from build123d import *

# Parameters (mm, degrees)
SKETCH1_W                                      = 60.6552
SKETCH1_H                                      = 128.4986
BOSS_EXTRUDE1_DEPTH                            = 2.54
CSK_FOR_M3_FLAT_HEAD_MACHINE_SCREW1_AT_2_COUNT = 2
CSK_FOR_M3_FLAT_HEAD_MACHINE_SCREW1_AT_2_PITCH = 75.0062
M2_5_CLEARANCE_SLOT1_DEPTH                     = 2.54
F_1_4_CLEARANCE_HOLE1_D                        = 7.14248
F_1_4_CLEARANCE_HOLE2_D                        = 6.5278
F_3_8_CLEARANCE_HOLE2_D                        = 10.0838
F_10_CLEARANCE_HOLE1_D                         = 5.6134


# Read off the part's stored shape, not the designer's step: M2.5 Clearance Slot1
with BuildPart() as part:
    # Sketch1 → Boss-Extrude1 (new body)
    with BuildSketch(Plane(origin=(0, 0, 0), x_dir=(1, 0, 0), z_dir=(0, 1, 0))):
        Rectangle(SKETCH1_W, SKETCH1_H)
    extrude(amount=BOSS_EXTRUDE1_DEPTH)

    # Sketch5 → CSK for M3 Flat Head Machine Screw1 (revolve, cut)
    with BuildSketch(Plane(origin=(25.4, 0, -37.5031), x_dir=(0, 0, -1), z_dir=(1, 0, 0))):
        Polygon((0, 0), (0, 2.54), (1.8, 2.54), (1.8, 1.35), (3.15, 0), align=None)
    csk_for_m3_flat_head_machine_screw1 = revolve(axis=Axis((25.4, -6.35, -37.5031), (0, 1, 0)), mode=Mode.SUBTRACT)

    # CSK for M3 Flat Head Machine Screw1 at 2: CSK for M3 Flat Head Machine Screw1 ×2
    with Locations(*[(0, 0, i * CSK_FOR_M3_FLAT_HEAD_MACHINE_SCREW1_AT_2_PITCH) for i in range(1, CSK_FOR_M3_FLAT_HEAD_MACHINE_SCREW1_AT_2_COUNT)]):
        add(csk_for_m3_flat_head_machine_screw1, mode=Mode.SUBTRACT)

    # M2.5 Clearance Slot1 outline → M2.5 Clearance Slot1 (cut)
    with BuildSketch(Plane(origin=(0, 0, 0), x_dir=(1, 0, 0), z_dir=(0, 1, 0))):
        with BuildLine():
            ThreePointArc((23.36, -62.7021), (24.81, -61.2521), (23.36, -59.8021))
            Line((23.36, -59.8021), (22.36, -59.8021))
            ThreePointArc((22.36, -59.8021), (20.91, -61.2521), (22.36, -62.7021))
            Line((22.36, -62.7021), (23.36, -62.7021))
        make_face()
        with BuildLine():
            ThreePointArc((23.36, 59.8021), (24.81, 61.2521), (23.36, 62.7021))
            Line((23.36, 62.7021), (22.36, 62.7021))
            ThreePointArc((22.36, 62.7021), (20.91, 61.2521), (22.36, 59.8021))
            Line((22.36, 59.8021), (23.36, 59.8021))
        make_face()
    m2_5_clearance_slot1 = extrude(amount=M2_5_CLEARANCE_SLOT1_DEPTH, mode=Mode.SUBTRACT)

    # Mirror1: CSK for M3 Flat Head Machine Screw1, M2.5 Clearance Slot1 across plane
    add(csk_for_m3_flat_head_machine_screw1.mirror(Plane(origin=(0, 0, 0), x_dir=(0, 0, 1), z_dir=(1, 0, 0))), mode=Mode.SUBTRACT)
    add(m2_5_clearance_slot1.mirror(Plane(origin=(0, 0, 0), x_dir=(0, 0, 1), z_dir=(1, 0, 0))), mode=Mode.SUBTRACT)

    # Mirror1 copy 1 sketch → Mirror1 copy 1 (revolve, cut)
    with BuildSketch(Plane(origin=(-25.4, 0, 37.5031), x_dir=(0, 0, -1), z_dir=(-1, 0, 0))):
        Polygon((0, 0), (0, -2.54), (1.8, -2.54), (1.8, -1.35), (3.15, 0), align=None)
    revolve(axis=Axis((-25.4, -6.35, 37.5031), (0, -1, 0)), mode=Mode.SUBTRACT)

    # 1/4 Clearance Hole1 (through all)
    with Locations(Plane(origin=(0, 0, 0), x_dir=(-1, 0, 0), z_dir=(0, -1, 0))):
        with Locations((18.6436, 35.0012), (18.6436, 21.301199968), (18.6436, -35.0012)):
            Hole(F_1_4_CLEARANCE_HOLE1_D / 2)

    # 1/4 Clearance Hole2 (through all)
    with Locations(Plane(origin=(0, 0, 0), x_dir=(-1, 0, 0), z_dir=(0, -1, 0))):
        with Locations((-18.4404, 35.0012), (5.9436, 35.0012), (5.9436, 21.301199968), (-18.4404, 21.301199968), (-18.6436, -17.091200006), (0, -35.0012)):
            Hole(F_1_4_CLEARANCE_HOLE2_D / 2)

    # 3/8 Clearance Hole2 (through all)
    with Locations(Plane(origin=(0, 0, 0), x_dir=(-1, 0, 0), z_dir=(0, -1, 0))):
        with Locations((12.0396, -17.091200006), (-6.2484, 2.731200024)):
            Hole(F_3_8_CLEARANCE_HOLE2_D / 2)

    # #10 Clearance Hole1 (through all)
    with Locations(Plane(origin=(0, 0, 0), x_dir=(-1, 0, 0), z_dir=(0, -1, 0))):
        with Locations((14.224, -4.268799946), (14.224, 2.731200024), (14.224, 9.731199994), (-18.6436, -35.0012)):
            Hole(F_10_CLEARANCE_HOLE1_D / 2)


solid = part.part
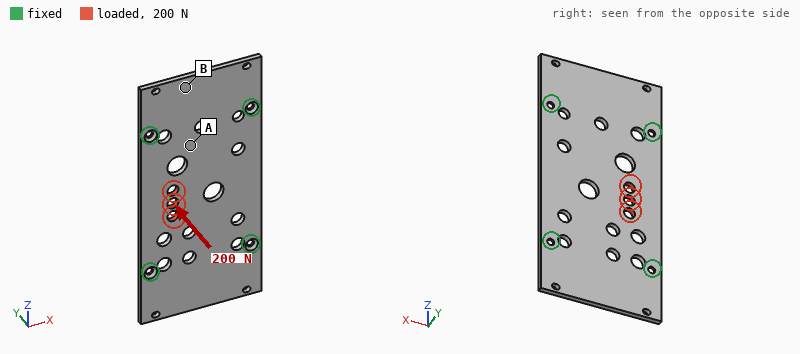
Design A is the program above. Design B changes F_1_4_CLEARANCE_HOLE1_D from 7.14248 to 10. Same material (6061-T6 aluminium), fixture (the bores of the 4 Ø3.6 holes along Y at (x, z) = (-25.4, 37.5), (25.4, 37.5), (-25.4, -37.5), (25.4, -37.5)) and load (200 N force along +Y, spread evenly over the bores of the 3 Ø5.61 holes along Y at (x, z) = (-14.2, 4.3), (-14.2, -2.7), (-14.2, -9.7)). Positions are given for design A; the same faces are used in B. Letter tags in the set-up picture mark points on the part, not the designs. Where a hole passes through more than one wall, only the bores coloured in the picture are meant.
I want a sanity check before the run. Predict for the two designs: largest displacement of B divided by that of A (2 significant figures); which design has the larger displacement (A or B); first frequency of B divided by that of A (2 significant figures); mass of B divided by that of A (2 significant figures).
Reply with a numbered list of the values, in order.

1. 1.1
2. B
3. 0.97
4. 0.98
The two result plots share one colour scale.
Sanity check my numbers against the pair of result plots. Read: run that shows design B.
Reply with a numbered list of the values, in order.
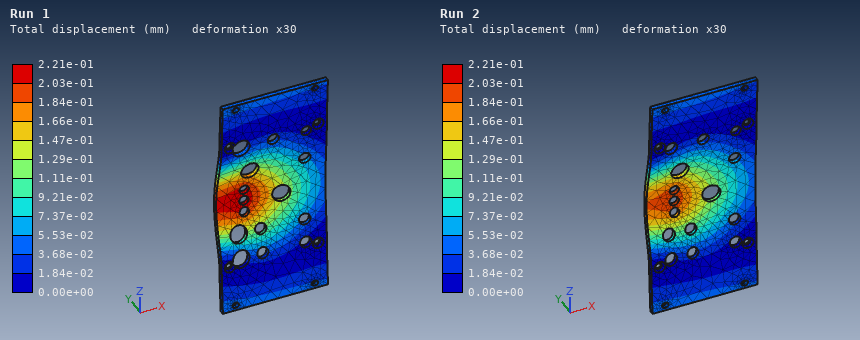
1. Run 1
